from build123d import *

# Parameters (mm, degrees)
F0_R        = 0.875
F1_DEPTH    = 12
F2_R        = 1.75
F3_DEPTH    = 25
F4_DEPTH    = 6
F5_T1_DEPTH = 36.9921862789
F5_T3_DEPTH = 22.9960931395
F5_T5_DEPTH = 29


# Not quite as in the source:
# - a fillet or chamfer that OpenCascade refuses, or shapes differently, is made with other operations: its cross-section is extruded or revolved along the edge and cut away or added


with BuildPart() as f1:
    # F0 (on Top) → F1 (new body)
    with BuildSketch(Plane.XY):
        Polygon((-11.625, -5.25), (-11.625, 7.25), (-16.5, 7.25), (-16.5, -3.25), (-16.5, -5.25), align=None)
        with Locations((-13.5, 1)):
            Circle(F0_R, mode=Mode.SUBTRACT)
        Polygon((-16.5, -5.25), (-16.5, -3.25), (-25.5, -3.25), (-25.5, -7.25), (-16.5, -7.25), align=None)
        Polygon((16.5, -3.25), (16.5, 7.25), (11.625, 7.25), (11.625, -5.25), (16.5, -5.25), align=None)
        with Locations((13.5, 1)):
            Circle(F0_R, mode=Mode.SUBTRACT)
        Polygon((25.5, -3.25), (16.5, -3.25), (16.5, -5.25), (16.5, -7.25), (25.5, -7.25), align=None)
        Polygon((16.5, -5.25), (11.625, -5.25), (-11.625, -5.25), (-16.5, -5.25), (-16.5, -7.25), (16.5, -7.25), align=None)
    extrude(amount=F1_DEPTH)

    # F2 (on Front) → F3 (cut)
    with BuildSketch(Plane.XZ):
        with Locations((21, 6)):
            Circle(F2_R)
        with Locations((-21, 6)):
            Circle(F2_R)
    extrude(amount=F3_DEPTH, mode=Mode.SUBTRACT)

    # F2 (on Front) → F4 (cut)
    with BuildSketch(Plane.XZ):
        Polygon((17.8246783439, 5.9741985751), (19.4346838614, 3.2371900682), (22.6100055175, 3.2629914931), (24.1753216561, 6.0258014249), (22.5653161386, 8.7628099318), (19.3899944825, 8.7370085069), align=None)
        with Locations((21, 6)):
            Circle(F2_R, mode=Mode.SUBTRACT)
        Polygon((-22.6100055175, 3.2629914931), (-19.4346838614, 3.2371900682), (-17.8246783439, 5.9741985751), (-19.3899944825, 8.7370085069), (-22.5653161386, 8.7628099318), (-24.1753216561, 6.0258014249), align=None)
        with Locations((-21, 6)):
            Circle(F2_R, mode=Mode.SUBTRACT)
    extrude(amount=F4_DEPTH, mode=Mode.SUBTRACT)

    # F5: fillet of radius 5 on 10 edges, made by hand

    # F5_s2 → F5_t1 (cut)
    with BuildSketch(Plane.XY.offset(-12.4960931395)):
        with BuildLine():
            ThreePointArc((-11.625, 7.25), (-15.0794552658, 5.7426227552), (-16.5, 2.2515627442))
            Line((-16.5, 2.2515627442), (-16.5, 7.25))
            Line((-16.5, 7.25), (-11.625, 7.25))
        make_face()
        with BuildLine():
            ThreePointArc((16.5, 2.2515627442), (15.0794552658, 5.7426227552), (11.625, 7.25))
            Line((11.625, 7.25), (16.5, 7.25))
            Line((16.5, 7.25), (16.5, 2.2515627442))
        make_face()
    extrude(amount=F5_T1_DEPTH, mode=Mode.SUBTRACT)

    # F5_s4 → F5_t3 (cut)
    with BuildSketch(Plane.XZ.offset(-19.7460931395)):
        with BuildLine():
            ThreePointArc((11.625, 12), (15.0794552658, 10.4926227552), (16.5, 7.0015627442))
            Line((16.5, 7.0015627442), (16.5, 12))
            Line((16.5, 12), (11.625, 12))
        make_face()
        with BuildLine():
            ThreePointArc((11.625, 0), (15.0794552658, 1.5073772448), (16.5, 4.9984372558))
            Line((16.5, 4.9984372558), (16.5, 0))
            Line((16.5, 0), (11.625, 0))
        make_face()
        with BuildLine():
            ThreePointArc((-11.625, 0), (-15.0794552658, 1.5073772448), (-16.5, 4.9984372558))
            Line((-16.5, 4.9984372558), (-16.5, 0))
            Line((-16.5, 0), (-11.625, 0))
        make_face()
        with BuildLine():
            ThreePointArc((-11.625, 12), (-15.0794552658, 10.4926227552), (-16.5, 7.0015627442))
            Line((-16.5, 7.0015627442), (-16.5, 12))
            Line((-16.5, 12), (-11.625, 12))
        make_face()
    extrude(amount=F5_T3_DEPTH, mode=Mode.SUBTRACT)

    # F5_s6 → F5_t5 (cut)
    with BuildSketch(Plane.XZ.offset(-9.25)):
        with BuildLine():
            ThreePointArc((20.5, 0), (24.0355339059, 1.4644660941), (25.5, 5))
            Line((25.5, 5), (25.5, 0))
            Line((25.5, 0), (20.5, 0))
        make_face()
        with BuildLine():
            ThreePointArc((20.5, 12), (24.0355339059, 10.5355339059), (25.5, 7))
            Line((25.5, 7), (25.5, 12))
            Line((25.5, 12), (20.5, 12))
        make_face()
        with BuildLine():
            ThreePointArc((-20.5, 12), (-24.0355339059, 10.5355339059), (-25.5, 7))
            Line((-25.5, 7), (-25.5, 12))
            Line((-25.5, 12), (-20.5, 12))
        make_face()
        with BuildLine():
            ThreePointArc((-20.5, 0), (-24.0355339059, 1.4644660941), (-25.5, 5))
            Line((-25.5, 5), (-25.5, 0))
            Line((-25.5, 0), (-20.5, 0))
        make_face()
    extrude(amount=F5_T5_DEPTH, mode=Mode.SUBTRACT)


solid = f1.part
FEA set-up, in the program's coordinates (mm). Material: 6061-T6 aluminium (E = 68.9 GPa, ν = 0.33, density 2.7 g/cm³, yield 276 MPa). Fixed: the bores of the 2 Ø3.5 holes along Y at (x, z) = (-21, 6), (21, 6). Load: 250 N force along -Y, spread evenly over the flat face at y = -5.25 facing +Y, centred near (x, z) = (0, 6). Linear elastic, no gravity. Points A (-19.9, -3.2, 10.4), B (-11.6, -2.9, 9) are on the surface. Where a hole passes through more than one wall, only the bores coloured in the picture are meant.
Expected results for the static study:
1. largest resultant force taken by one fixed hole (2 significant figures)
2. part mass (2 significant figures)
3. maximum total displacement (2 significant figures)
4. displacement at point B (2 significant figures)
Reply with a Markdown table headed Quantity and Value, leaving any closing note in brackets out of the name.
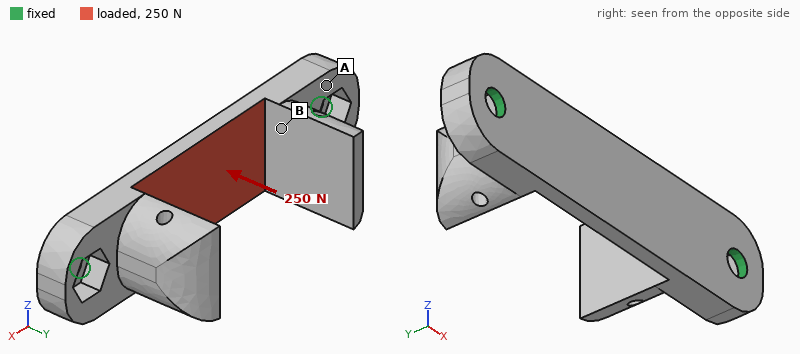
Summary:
| Quantity | Value |
|---|---|
| largest resultant force taken by one fixed hole | 130 N |
| part mass | 6.8 g |
| maximum total displacement | 85 µm |
| displacement at point B | 40 µm |
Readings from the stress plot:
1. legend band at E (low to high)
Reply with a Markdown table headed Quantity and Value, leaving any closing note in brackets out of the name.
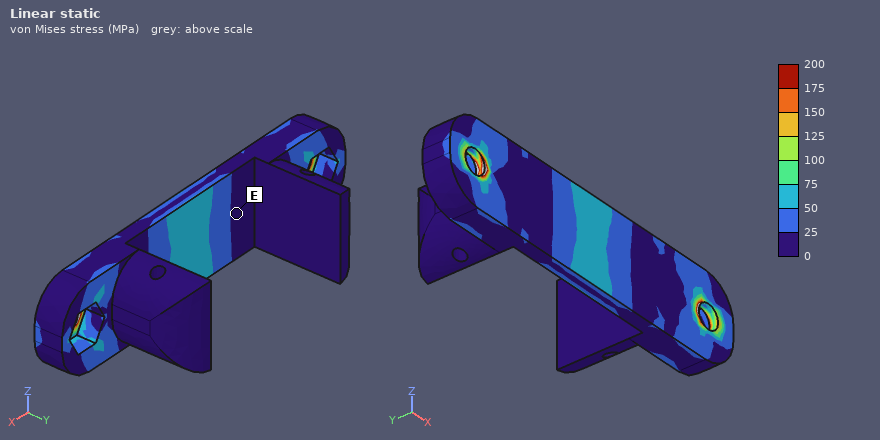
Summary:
| Quantity | Value |
|---|---|
| legend band at E | 0 to 25 MPa |
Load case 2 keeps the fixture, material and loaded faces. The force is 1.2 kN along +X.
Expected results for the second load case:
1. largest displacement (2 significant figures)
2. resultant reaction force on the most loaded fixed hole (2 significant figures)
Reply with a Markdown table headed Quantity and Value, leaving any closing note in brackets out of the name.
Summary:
| Quantity | Value |
|---|---|
| largest displacement | 7.0 µm |
| resultant reaction force on the most loaded fixed hole | 600 N |
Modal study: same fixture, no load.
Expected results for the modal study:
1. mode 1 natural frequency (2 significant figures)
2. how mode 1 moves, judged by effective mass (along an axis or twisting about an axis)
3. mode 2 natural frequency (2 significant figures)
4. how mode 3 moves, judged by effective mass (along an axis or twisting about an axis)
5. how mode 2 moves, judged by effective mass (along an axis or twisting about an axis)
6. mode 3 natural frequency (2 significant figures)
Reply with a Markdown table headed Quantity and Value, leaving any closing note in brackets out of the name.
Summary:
| Quantity | Value |
|---|---|
| mode 1 natural frequency | 5400 Hz |
| how mode 1 moves, judged by effective mass | along Y |
| mode 2 natural frequency | 8100 Hz |
| how mode 3 moves, judged by effective mass | along X |
| how mode 2 moves, judged by effective mass | along Z |
| mode 3 natural frequency | 8700 Hz |
